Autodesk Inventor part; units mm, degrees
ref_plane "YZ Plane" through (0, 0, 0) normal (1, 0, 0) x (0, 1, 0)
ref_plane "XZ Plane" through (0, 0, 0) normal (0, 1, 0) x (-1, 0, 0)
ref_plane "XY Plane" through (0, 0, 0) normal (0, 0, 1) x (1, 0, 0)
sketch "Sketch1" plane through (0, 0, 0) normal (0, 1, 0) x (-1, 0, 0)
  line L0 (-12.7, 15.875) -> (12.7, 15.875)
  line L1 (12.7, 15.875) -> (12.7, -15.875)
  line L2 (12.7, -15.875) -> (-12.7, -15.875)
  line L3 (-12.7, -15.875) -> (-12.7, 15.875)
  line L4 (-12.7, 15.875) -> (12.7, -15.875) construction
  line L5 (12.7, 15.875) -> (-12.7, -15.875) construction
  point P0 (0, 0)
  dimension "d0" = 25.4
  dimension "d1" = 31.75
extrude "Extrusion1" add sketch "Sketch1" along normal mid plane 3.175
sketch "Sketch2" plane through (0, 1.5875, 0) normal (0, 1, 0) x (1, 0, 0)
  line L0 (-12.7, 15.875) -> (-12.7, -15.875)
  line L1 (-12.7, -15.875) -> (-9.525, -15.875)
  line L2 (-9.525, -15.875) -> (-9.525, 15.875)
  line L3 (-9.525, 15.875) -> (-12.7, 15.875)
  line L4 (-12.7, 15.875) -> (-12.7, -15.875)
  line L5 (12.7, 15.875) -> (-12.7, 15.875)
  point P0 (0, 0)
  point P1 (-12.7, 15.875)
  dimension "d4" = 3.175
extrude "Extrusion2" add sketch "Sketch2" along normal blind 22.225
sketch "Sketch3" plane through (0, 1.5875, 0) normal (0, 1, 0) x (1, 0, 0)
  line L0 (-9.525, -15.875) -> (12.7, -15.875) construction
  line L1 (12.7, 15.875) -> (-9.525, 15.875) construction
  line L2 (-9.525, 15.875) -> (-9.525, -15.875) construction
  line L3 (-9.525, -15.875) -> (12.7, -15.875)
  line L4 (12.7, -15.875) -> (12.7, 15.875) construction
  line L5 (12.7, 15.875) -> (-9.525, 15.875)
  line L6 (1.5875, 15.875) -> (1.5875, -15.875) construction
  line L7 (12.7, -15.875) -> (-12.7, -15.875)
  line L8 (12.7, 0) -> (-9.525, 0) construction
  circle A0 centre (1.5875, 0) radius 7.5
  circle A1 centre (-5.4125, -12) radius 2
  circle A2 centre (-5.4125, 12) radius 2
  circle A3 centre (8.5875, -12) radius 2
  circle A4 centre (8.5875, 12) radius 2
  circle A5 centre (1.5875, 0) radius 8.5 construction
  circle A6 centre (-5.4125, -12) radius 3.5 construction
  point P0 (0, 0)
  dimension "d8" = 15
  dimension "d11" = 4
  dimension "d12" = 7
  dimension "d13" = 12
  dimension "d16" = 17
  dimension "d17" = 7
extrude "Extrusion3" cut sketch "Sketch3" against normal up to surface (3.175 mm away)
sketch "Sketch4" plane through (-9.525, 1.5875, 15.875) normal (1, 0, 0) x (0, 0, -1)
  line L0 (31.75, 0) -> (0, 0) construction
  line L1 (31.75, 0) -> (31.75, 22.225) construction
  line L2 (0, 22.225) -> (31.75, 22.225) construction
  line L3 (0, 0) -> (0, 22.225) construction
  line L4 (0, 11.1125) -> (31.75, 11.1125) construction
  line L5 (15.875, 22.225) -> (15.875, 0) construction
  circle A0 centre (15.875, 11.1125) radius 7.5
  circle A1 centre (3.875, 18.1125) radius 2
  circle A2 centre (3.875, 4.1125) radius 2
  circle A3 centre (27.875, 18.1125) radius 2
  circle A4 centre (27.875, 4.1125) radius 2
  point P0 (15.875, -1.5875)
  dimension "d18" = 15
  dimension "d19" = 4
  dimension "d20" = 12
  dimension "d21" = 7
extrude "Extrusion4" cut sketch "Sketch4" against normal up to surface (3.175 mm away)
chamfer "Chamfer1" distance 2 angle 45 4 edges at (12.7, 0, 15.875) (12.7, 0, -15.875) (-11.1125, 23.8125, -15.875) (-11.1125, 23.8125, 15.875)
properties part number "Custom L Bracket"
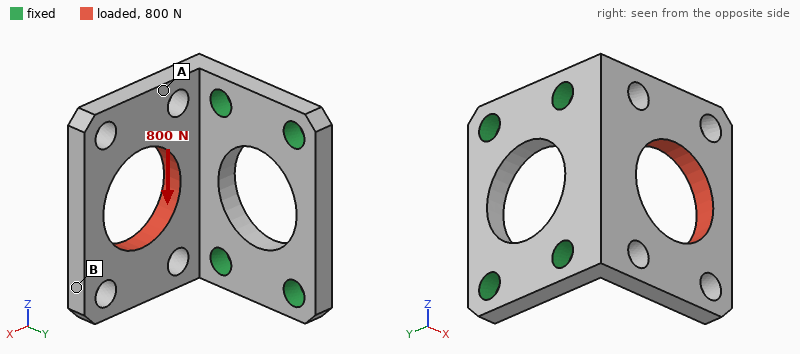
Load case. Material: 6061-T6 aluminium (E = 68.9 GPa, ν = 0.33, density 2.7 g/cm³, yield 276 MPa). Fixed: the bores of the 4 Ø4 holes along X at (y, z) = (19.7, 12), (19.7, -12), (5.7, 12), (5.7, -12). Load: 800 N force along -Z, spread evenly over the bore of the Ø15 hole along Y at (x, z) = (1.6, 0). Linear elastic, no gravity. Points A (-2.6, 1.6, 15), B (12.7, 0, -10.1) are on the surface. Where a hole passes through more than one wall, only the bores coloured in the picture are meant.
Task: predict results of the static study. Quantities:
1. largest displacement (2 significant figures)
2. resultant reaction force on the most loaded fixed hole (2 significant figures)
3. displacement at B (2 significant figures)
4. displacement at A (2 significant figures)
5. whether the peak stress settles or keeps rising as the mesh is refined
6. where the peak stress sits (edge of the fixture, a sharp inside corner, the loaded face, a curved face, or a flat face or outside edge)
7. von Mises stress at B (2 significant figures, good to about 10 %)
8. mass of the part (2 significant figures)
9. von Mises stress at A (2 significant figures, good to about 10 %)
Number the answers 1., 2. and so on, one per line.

1. 46 µm
2. 570 N
3. 42 µm
4. 23 µm
5. keeps rising
6. edge of the fixture
7. 16 MPa
8. 9.0 g
9. 38 MPa
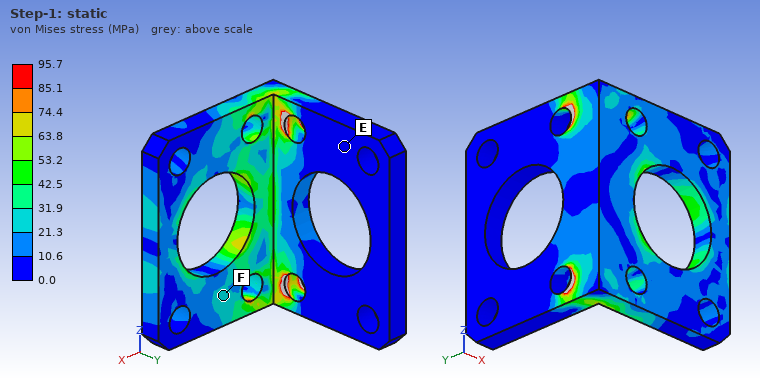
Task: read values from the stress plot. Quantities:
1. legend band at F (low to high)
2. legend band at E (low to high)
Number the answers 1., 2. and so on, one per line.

1. 21.3 to 31.9 MPa
2. 0.0 to 10.6 MPa
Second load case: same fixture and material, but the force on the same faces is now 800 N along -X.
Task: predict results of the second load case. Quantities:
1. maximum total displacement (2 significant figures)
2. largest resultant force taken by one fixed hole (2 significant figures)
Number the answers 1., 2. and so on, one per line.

1. 57 µm
2. 420 N
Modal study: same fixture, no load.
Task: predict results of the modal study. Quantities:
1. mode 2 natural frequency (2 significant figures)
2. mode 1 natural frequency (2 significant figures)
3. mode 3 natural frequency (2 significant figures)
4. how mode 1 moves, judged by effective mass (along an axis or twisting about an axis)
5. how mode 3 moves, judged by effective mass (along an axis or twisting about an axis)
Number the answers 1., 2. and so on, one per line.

1. 6800 Hz
2. 3400 Hz
3. 13 kHz
4. along Y
5. along Z
